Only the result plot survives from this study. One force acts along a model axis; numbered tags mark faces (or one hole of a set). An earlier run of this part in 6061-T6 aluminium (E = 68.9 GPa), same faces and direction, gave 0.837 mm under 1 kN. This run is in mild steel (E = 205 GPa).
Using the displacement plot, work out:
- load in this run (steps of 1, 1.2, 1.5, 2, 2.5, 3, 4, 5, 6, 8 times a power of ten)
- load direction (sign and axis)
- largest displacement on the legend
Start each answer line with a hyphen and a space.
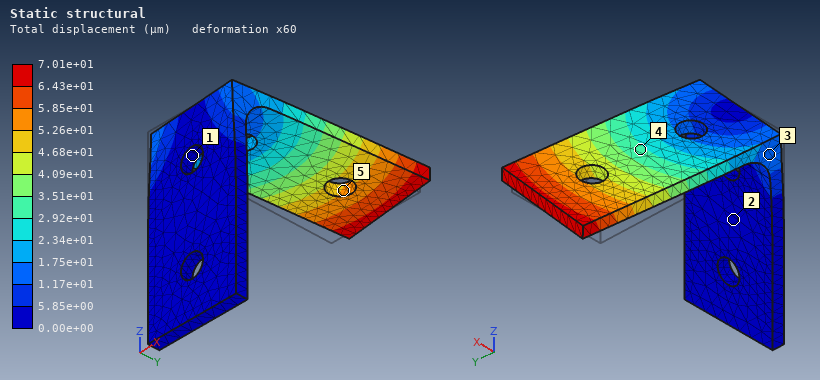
- 250 N
- +X
- 7.01e+01 µm
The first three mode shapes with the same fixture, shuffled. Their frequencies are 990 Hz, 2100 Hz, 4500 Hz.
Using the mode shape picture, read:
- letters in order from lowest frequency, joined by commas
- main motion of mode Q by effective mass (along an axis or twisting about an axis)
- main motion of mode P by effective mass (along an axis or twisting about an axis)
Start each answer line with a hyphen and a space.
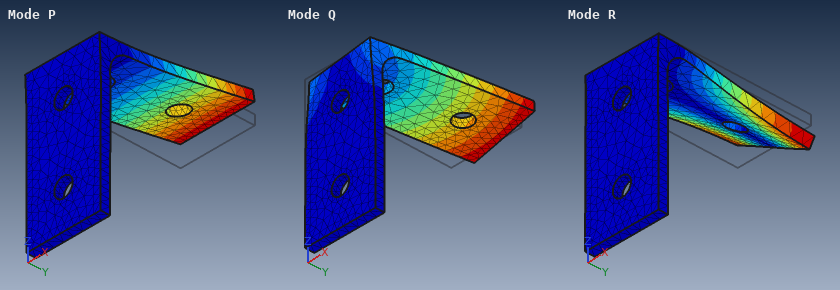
- P, Q, R
- along X
- along Z
